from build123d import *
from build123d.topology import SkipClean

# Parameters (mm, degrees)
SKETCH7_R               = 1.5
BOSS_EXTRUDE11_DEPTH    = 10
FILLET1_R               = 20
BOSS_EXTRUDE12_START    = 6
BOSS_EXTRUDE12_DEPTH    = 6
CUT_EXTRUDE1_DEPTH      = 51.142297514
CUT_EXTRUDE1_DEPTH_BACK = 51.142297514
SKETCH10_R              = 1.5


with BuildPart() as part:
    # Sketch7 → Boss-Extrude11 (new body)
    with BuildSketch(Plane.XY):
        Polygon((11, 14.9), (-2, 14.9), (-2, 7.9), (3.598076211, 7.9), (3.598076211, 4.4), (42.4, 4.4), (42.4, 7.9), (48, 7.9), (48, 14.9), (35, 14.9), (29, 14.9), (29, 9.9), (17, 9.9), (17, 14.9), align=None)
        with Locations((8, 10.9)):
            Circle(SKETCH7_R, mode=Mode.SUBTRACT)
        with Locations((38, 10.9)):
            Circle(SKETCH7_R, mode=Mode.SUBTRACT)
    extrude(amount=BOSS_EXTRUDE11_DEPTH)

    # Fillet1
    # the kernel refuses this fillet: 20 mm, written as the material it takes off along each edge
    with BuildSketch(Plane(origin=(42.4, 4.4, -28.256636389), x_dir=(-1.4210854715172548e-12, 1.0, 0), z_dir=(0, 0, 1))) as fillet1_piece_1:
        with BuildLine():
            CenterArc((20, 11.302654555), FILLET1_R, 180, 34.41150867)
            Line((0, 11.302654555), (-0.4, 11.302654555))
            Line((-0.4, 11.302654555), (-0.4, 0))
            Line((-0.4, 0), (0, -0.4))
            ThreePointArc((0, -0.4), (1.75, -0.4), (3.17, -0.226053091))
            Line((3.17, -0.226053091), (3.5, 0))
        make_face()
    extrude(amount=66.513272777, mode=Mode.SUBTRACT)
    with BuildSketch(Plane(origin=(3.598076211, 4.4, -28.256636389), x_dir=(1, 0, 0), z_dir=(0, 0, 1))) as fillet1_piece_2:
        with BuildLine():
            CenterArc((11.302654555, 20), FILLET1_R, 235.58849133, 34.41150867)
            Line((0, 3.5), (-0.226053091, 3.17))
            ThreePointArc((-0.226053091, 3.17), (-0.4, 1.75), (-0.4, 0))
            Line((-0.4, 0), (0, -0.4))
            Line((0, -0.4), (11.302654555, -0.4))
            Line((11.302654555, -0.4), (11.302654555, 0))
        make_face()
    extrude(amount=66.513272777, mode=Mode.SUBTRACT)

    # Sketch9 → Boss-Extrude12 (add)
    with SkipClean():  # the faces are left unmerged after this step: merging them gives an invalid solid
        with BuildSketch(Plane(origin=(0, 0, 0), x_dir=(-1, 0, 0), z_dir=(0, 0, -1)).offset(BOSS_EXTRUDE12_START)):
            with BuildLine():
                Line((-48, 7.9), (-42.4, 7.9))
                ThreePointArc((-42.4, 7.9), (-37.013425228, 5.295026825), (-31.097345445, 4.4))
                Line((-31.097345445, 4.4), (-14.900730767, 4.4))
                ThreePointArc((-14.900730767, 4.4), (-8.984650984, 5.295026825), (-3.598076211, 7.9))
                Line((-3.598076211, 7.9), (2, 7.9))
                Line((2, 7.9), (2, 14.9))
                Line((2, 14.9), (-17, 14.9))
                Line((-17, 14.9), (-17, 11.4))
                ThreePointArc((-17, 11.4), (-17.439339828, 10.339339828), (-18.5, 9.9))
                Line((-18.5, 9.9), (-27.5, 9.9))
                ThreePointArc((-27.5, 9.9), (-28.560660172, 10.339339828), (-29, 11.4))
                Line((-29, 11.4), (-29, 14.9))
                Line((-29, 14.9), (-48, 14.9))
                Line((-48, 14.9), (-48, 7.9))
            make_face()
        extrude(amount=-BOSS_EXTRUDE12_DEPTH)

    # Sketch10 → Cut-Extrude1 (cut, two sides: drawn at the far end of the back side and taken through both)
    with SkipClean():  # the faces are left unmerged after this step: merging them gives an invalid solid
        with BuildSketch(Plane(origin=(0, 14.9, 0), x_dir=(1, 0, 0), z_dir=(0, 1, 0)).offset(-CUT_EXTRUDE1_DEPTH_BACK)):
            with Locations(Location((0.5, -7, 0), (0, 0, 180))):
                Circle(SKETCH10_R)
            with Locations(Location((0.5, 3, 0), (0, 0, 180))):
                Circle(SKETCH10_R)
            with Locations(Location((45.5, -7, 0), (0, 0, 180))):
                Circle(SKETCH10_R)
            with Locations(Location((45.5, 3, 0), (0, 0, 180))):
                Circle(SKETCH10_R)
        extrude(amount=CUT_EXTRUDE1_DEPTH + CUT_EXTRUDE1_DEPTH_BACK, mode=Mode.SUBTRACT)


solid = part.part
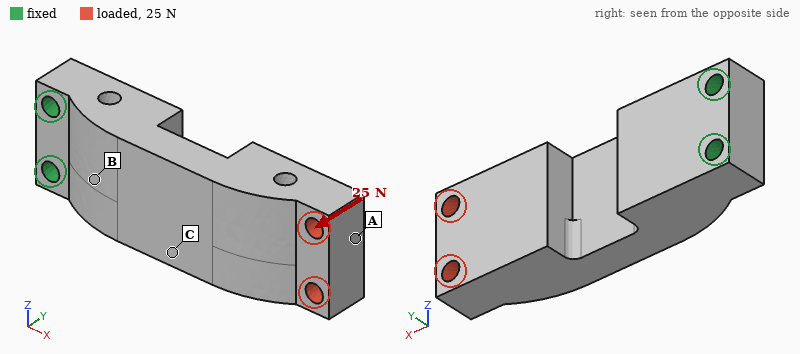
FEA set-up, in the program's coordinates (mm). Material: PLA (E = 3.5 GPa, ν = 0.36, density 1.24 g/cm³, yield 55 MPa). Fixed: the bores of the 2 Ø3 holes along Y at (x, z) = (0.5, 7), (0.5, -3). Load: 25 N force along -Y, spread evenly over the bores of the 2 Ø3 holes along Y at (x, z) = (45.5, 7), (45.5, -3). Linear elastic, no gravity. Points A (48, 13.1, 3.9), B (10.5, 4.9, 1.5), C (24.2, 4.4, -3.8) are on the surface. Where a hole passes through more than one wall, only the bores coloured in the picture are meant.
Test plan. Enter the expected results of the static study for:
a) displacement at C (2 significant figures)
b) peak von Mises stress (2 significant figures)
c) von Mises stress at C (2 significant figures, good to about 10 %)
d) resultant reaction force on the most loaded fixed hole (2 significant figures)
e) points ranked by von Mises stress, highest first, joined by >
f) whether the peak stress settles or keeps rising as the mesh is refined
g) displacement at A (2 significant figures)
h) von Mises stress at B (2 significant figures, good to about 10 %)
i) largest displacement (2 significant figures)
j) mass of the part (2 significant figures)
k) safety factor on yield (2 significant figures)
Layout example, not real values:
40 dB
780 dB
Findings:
0.15 mm
19 MPa
6.7 MPa
13 N
C > B > A
settles
0.55 mm
3.3 MPa
0.55 mm
7.5 g
2.8
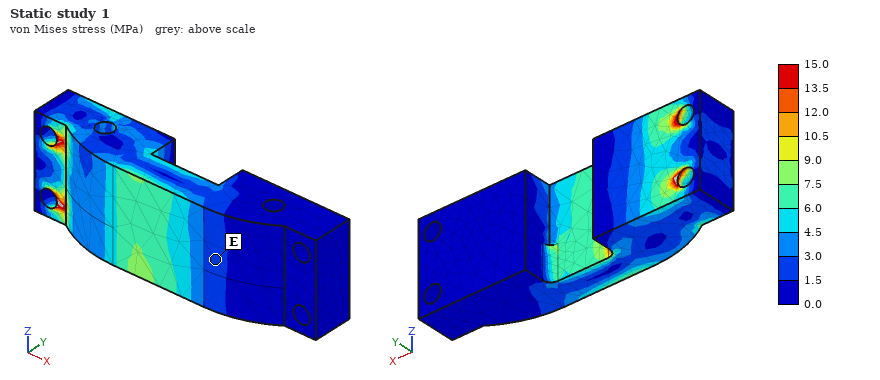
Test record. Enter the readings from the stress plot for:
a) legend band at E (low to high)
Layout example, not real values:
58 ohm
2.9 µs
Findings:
1.5 to 3.0 MPa
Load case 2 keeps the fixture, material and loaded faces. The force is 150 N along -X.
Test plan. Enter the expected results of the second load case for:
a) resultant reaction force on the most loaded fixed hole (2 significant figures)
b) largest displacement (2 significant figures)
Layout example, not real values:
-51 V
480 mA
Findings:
76 N
0.36 mm
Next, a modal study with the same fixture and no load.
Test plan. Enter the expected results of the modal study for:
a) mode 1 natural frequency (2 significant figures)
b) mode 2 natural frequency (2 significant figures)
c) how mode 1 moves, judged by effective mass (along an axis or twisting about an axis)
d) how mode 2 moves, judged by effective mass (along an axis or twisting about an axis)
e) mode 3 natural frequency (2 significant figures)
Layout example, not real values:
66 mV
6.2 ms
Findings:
820 Hz
1600 Hz
along Y
along Z
3500 Hz
